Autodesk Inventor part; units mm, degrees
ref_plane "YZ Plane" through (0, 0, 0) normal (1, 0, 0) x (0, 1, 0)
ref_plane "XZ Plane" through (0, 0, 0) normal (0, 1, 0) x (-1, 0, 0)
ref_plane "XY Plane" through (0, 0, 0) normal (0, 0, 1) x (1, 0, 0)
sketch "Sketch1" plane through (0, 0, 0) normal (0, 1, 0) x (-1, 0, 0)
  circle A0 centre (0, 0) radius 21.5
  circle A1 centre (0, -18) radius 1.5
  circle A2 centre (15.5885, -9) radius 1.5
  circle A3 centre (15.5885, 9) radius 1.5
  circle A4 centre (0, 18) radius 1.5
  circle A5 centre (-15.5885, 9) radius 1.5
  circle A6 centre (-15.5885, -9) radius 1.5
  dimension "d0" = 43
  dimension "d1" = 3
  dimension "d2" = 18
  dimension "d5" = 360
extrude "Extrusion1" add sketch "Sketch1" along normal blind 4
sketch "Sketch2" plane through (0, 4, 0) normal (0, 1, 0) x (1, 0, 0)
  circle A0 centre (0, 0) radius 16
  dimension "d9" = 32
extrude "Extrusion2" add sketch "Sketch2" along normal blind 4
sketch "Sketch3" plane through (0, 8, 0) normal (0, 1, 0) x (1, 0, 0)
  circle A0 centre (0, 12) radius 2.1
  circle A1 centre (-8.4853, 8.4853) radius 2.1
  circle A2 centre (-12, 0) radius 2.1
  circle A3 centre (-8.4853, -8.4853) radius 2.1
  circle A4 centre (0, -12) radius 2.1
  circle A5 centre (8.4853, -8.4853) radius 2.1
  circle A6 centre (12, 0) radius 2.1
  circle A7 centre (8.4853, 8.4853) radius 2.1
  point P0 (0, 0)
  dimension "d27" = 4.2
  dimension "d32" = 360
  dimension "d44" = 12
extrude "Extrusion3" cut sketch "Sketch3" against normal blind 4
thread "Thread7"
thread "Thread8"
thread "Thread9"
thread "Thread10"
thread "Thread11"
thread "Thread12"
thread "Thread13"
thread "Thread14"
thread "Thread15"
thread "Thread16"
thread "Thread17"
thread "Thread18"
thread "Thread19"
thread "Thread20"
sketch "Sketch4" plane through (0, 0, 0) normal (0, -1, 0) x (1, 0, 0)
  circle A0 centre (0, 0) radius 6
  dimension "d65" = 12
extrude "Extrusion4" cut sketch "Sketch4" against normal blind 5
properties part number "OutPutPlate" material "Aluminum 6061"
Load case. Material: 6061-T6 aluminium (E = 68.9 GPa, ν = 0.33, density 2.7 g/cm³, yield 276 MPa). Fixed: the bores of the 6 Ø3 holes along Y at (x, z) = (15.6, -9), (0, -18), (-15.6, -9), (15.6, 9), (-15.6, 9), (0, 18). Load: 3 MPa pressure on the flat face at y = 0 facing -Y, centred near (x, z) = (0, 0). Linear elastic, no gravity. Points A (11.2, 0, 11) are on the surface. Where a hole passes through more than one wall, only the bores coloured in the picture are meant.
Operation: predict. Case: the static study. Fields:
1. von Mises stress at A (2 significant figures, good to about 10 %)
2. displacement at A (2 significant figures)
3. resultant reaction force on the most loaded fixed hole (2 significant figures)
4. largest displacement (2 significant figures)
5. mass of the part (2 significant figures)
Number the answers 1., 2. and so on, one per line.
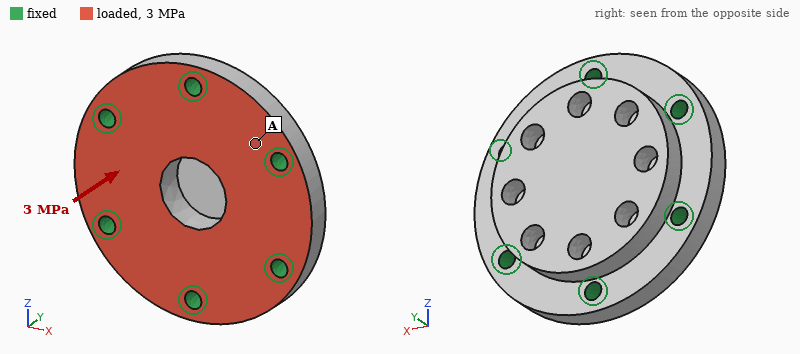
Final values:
1. 10 MPa
2. 2.3 µm
3. 660 N
4. 4.8 µm
5. 21 g
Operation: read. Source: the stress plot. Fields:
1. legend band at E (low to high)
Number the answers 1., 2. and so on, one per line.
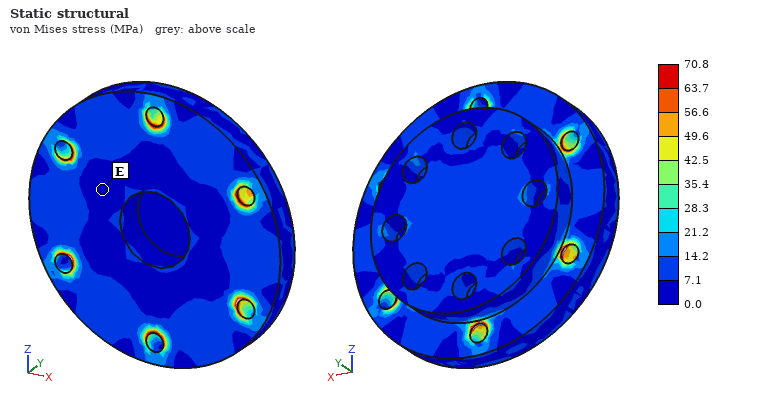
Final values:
1. 0.0 to 7.1 MPa
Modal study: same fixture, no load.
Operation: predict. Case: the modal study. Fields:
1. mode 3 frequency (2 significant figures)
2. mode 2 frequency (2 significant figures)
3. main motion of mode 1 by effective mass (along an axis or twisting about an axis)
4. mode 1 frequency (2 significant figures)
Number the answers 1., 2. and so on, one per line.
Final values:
1. 46 kHz
2. 46 kHz
3. along Y
4. 31 kHz
